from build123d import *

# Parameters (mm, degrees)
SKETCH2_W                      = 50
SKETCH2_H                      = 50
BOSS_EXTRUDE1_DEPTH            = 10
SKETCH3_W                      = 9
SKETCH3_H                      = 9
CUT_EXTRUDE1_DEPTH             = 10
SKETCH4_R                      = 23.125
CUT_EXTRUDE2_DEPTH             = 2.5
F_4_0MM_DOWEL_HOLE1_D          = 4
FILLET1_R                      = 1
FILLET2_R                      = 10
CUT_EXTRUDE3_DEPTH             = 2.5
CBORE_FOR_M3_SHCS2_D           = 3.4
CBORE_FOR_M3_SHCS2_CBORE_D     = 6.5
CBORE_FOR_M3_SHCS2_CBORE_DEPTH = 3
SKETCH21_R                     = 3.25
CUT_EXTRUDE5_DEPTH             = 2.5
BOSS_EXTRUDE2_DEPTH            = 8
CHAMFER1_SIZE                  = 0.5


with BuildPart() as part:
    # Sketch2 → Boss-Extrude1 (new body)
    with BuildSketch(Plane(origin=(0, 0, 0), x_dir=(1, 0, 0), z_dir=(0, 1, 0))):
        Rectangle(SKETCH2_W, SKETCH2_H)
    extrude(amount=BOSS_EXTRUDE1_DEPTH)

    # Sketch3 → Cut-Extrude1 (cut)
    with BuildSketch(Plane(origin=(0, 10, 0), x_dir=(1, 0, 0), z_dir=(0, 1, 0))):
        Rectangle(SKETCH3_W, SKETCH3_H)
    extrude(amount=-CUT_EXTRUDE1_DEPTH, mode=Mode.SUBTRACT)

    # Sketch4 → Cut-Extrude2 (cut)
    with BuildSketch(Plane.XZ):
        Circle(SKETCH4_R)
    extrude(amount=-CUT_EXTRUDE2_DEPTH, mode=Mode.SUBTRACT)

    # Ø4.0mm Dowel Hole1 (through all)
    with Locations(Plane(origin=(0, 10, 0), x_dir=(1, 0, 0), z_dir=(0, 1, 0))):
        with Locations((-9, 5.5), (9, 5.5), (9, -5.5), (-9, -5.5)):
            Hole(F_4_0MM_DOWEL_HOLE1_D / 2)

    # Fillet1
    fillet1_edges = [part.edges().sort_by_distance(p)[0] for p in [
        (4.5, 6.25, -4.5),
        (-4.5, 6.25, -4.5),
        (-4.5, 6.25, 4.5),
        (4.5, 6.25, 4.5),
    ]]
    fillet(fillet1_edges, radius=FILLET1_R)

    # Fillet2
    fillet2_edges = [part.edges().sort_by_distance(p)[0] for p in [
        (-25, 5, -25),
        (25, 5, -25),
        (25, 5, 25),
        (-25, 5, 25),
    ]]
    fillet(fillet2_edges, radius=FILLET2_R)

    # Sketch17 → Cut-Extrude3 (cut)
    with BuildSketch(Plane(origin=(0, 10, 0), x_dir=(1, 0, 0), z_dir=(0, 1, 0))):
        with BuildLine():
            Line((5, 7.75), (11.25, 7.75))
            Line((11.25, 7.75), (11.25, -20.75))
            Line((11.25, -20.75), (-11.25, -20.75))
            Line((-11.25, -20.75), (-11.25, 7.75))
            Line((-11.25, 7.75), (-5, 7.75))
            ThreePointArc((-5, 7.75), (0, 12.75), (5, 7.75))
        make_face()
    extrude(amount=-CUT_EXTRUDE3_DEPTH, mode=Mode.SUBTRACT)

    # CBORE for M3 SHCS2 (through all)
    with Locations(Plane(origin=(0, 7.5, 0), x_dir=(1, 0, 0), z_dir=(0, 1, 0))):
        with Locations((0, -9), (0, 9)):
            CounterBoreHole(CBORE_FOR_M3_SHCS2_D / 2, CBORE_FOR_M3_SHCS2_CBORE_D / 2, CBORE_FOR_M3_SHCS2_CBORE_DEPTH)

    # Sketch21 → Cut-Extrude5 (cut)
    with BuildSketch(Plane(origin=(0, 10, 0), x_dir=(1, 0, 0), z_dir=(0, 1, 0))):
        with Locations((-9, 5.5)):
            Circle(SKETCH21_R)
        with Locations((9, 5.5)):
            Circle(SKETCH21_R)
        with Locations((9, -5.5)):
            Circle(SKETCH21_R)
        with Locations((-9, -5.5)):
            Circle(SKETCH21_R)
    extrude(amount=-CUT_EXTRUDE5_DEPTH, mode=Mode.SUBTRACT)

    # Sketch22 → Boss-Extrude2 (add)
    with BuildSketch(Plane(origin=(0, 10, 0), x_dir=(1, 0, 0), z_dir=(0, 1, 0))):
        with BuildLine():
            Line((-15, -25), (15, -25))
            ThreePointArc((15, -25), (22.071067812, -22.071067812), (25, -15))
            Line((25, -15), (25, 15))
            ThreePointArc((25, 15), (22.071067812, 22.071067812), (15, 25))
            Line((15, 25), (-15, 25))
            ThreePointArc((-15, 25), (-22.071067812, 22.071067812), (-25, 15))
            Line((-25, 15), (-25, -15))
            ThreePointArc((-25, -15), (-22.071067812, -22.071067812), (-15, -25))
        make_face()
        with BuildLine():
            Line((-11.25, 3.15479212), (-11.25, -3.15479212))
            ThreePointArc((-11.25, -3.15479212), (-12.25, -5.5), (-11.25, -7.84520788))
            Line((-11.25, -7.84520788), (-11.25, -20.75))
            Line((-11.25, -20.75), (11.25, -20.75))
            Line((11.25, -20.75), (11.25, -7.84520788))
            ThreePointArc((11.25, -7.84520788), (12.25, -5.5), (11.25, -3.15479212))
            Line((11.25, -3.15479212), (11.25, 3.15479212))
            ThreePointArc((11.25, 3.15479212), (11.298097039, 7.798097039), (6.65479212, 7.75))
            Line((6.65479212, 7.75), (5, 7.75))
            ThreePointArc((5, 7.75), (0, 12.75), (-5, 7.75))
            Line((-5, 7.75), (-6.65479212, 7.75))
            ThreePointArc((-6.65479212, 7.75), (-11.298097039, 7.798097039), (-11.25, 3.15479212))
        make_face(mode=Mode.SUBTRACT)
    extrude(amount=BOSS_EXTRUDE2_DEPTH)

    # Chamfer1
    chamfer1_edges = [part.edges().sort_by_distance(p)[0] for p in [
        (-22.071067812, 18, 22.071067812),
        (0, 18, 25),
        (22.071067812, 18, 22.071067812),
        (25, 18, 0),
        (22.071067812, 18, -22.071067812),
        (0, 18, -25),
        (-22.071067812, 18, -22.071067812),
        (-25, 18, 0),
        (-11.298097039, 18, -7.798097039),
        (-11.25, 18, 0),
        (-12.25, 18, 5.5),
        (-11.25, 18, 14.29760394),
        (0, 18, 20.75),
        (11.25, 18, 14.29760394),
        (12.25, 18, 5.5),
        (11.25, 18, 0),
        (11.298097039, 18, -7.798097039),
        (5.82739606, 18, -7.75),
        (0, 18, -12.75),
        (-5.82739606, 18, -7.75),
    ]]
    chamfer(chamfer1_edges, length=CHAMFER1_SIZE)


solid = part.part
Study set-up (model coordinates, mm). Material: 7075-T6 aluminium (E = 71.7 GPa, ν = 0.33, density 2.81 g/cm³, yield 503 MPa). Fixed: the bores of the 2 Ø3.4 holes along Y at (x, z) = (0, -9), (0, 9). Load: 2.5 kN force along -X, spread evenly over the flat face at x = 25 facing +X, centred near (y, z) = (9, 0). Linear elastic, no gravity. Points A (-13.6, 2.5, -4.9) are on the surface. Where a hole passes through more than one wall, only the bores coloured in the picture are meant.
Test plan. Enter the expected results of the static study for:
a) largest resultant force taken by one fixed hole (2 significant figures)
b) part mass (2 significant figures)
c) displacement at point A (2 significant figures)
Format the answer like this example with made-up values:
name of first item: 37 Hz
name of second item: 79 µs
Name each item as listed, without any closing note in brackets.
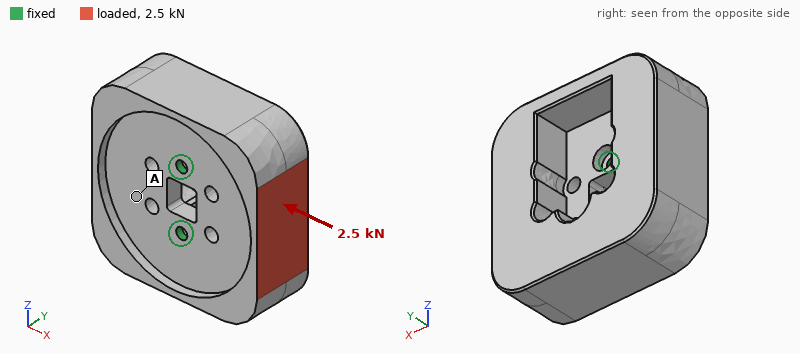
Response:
largest resultant force taken by one fixed hole: 1.3 kN
part mass: 87 g
displacement at point A: 0.098 mm
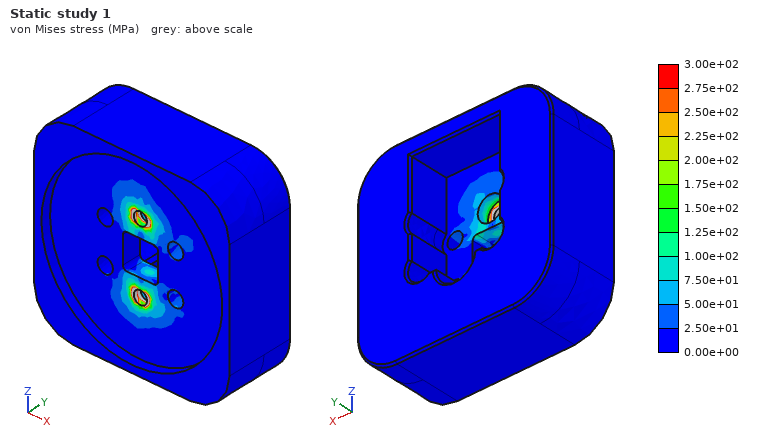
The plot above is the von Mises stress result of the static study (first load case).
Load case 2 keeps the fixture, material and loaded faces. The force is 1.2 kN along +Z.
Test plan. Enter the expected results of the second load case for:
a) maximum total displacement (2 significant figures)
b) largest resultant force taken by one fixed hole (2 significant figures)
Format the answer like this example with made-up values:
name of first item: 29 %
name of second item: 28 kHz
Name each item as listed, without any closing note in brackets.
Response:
maximum total displacement: 29 µm
largest resultant force taken by one fixed hole: 1.6 kN
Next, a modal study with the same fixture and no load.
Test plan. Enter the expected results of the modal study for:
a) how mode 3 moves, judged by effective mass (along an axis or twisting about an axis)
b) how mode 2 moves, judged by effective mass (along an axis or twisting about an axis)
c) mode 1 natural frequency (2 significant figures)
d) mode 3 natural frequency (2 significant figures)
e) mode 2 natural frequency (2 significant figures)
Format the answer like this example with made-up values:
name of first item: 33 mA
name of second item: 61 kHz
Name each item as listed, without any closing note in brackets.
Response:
how mode 3 moves, judged by effective mass: twisting about Y
how mode 2 moves, judged by effective mass: along Z
mode 1 natural frequency: 1300 Hz
mode 3 natural frequency: 5300 Hz
mode 2 natural frequency: 4100 Hz
